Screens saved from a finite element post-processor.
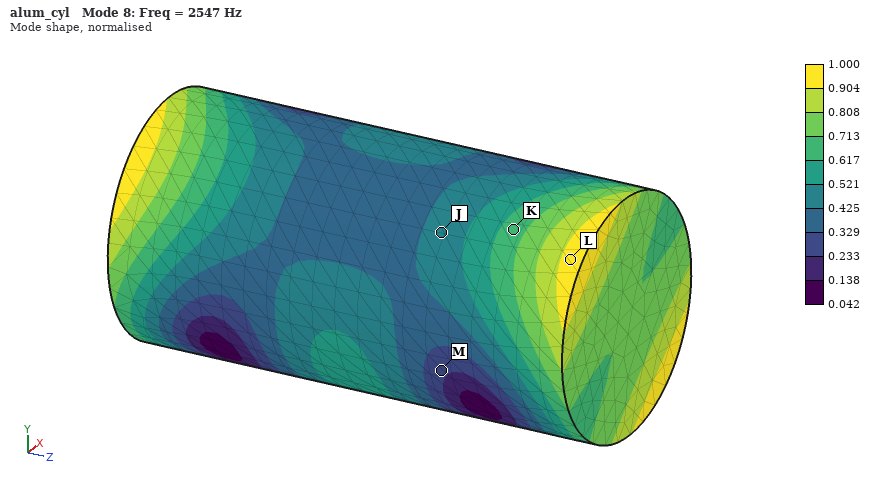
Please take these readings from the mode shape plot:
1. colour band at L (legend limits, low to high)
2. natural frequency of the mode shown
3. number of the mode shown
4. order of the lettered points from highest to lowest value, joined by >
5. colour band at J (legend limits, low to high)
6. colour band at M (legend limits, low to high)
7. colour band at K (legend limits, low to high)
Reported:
0.904 to 1.000
2547 Hz
8
L > K > J > M
0.425 to 0.521
0.233 to 0.329
0.617 to 0.713
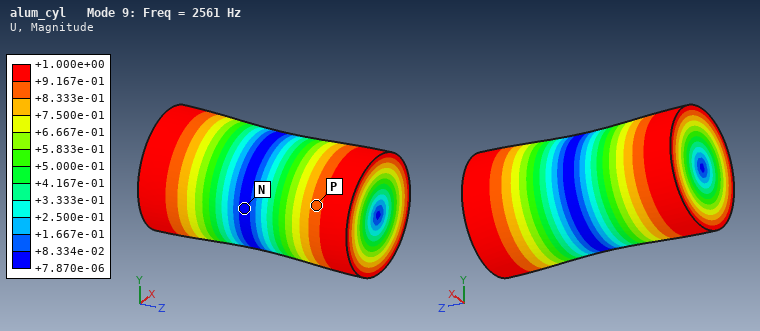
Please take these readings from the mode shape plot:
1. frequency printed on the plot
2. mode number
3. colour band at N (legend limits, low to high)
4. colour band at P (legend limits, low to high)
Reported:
2561 Hz
9
+7.870e-06 to +8.334e-02
+8.333e-01 to +9.167e-01
